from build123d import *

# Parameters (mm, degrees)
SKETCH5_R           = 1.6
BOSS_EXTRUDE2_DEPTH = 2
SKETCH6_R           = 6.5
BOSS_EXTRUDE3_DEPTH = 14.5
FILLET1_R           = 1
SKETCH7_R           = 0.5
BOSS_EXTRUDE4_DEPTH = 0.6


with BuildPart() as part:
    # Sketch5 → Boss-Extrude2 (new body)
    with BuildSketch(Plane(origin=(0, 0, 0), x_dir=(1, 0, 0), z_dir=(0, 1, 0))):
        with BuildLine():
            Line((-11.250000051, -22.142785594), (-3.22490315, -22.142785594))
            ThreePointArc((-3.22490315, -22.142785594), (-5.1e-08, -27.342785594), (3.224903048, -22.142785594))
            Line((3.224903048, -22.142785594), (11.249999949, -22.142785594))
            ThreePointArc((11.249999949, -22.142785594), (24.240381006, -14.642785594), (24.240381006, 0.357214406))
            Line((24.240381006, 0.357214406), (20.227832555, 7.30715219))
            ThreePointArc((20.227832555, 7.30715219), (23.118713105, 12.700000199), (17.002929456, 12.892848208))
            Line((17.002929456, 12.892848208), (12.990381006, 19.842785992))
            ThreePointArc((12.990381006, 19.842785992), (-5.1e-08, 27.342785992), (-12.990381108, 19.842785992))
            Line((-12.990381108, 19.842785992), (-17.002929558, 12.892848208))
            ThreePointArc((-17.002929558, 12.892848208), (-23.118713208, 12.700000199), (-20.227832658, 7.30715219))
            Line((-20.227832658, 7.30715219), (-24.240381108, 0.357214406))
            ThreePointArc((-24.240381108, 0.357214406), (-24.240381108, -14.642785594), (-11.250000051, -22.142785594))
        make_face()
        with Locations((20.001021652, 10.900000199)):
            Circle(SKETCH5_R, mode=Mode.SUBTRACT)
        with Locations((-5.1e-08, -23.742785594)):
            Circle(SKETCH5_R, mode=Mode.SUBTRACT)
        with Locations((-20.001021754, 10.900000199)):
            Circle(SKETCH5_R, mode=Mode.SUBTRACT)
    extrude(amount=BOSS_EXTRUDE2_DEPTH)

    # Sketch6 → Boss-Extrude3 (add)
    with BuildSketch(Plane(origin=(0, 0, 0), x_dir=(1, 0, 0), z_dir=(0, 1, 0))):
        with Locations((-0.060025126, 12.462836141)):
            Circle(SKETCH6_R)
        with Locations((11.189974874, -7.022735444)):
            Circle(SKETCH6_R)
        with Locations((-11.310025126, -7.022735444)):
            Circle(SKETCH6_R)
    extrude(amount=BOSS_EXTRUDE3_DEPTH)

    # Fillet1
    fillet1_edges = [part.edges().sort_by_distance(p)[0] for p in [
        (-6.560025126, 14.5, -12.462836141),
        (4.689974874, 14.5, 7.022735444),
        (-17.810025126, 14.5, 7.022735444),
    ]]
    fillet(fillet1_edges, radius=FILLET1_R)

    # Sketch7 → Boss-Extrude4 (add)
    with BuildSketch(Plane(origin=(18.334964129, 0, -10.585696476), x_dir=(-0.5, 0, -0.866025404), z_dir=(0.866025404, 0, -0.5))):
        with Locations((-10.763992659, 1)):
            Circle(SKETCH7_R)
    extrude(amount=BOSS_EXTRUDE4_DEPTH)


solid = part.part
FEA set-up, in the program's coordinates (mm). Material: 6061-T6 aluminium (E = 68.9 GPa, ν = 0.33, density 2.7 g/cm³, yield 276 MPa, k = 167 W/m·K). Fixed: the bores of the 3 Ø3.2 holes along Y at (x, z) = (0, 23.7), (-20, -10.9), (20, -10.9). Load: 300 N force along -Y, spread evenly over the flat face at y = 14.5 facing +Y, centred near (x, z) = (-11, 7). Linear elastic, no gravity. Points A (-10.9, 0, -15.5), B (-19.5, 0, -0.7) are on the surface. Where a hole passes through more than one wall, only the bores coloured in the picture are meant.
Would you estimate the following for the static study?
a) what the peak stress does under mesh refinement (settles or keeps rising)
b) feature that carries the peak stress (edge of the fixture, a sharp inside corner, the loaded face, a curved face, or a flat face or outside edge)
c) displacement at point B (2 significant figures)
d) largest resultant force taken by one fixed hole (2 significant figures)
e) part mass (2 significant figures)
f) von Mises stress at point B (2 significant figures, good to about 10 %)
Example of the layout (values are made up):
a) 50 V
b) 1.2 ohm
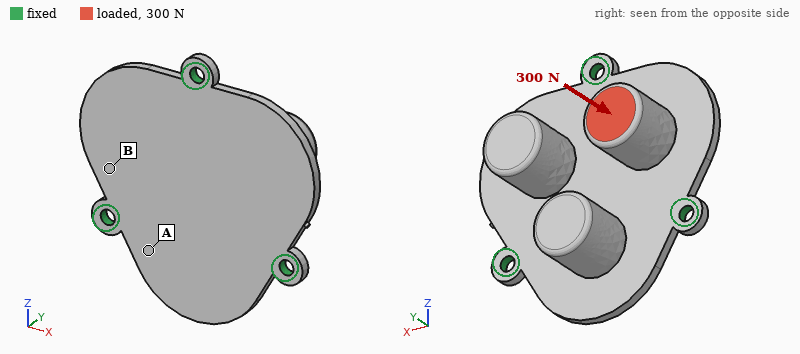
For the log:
a) keeps rising
b) edge of the fixture
c) 0.056 mm
d) 160 N
e) 24 g
f) 36 MPa
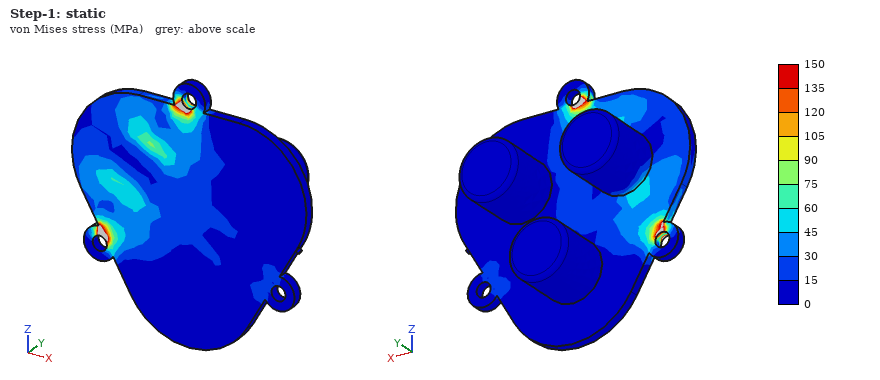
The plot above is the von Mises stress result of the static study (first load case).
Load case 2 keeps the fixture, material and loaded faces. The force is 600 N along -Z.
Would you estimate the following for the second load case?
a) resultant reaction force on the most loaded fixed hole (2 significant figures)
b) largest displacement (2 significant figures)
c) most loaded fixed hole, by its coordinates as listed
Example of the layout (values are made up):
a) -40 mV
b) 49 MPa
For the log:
a) 390 N
b) 0.25 mm
c) (0, 23.7)
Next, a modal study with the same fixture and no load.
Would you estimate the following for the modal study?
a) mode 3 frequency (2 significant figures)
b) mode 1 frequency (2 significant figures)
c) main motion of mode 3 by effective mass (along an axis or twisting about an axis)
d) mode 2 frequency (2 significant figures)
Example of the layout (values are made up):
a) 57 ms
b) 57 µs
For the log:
a) 3600 Hz
b) 3100 Hz
c) along Y
d) 3100 Hz
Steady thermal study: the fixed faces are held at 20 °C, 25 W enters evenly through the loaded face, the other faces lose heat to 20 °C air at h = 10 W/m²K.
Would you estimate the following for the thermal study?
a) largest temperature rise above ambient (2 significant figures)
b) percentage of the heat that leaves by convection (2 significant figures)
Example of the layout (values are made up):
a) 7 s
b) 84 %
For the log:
a) 49 K
b) 4.3 %
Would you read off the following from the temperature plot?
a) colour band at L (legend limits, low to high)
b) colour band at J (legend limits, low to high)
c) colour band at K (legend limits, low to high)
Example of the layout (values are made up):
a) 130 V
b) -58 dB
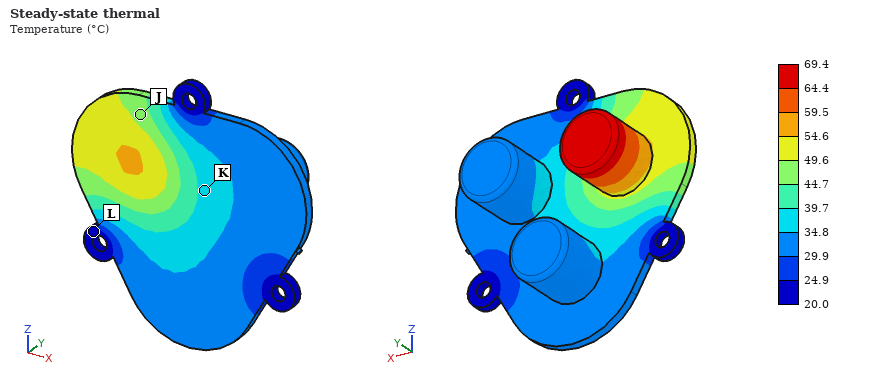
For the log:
a) 20.0 to 24.9 °C
b) 44.7 to 49.6 °C
c) 34.8 to 39.7 °C
